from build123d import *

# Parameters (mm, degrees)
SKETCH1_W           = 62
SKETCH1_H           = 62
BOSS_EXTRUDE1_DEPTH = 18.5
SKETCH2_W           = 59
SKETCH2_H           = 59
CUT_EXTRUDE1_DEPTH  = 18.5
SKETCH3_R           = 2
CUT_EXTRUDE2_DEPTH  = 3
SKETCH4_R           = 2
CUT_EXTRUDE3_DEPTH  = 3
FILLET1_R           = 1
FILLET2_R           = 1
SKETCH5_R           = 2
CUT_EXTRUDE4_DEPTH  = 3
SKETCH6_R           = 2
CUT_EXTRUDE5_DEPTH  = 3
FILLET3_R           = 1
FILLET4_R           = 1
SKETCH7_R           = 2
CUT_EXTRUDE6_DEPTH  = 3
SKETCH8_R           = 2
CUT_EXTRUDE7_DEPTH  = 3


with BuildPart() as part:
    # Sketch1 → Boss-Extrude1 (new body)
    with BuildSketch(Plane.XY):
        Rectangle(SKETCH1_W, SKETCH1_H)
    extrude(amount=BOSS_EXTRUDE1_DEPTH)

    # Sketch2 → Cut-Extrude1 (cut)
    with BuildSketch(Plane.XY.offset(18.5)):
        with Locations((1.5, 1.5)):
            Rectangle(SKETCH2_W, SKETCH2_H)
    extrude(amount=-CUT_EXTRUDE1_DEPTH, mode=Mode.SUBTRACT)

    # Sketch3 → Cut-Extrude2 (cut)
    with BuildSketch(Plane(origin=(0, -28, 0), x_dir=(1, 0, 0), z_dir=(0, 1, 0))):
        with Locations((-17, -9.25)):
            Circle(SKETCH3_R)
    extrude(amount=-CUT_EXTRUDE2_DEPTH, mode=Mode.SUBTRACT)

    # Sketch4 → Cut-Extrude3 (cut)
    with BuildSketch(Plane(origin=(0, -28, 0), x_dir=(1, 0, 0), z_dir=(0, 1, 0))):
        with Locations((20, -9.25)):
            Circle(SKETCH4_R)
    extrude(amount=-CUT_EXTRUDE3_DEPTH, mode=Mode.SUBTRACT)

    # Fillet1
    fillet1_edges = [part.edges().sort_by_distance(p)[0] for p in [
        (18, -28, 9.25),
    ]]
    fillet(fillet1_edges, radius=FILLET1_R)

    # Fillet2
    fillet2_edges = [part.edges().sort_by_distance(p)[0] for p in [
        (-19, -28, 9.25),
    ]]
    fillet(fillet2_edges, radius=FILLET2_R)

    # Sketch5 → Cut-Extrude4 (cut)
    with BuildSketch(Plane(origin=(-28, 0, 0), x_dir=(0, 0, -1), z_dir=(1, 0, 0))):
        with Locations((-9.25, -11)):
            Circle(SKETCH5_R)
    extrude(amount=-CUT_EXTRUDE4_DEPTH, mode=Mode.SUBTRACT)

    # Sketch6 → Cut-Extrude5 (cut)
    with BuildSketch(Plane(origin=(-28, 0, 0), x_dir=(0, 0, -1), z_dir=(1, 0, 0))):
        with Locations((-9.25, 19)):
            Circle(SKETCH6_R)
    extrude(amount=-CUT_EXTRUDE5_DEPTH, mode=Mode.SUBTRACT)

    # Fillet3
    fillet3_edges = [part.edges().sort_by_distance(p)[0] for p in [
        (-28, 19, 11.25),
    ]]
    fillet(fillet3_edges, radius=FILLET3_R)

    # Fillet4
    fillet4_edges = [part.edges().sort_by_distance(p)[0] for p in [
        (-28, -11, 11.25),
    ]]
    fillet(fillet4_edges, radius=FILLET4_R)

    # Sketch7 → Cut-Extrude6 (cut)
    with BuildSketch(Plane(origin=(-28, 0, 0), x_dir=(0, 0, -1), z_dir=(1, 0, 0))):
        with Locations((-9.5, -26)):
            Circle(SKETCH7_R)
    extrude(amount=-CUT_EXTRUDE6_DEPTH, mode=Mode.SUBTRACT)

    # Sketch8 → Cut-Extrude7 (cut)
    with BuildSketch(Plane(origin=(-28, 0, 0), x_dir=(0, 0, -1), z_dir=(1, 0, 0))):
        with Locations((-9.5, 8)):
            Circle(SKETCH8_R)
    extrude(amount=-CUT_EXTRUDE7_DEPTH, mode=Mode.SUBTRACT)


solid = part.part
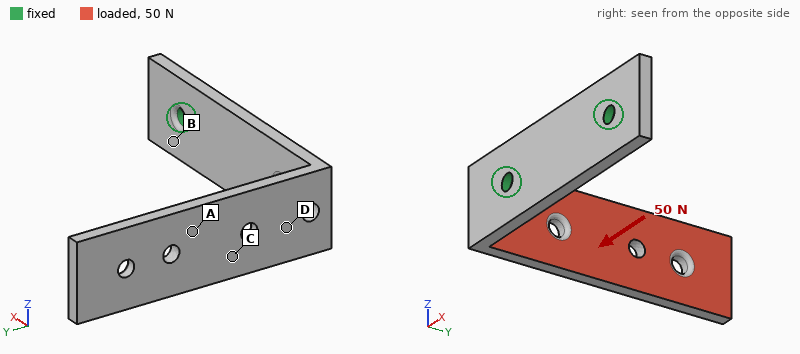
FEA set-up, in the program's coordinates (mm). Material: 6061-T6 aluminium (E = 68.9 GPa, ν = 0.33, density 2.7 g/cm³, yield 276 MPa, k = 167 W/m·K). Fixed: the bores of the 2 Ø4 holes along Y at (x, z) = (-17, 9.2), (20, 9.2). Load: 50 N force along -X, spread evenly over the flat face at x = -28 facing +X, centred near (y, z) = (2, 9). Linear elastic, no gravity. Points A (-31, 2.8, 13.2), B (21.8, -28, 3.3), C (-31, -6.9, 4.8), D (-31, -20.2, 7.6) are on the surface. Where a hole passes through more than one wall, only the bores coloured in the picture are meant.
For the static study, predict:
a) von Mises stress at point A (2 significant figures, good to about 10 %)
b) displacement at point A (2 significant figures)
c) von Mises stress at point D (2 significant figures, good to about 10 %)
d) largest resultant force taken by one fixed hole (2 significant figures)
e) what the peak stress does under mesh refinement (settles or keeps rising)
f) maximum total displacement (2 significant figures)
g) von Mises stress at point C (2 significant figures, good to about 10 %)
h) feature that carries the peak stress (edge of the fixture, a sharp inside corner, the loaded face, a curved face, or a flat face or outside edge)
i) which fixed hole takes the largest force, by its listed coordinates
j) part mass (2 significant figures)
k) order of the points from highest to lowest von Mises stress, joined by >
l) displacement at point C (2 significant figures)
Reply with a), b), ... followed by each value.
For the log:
a) 13 MPa
b) 0.43 mm
c) 34 MPa
d) 36 N
e) keeps rising
f) 0.94 mm
g) 24 MPa
h) edge of the fixture
i) (20, 9.2)
j) 17 g
k) D > C > A > B
l) 0.27 mm
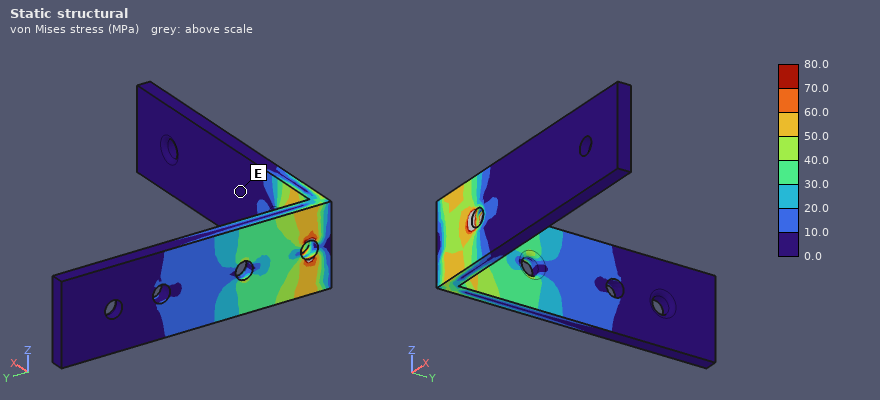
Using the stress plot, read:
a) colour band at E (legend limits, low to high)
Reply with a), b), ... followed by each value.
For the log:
a) 0.0 to 10.0 MPa
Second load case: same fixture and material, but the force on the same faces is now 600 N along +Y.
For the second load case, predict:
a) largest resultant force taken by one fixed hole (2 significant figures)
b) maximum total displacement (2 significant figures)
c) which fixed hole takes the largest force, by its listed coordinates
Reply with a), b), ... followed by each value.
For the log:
a) 640 N
b) 0.44 mm
c) (-17, 9.2)
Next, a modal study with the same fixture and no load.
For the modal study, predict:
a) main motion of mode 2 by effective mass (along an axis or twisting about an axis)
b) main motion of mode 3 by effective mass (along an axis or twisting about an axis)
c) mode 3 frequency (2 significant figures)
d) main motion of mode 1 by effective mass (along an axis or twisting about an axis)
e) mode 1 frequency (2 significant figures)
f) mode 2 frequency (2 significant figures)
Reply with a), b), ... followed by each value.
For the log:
a) along Z
b) along Y
c) 3000 Hz
d) along X
e) 490 Hz
f) 900 Hz
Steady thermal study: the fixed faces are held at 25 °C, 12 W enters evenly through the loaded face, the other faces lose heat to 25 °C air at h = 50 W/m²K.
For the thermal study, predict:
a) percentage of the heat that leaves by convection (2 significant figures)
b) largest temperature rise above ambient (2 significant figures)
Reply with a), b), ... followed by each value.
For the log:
a) 26 %
b) 44 K
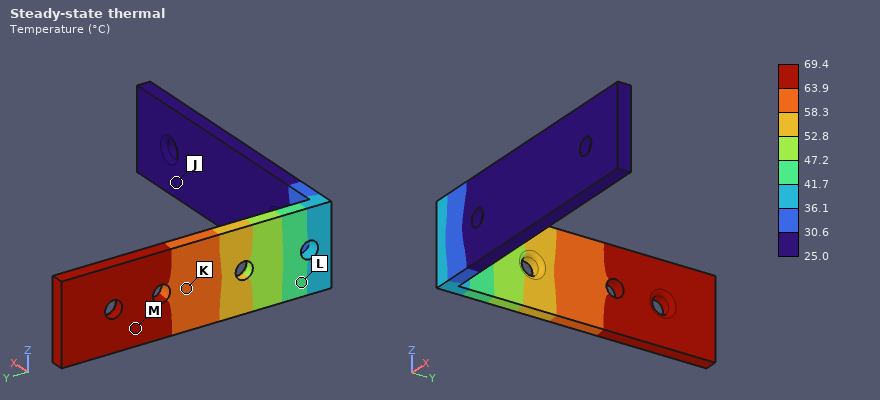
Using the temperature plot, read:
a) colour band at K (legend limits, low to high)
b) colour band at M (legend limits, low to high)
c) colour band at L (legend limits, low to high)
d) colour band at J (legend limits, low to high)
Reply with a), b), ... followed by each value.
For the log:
a) 58.3 to 63.9 °C
b) 63.9 to 69.4 °C
c) 41.7 to 47.2 °C
d) 25.0 to 30.6 °C
